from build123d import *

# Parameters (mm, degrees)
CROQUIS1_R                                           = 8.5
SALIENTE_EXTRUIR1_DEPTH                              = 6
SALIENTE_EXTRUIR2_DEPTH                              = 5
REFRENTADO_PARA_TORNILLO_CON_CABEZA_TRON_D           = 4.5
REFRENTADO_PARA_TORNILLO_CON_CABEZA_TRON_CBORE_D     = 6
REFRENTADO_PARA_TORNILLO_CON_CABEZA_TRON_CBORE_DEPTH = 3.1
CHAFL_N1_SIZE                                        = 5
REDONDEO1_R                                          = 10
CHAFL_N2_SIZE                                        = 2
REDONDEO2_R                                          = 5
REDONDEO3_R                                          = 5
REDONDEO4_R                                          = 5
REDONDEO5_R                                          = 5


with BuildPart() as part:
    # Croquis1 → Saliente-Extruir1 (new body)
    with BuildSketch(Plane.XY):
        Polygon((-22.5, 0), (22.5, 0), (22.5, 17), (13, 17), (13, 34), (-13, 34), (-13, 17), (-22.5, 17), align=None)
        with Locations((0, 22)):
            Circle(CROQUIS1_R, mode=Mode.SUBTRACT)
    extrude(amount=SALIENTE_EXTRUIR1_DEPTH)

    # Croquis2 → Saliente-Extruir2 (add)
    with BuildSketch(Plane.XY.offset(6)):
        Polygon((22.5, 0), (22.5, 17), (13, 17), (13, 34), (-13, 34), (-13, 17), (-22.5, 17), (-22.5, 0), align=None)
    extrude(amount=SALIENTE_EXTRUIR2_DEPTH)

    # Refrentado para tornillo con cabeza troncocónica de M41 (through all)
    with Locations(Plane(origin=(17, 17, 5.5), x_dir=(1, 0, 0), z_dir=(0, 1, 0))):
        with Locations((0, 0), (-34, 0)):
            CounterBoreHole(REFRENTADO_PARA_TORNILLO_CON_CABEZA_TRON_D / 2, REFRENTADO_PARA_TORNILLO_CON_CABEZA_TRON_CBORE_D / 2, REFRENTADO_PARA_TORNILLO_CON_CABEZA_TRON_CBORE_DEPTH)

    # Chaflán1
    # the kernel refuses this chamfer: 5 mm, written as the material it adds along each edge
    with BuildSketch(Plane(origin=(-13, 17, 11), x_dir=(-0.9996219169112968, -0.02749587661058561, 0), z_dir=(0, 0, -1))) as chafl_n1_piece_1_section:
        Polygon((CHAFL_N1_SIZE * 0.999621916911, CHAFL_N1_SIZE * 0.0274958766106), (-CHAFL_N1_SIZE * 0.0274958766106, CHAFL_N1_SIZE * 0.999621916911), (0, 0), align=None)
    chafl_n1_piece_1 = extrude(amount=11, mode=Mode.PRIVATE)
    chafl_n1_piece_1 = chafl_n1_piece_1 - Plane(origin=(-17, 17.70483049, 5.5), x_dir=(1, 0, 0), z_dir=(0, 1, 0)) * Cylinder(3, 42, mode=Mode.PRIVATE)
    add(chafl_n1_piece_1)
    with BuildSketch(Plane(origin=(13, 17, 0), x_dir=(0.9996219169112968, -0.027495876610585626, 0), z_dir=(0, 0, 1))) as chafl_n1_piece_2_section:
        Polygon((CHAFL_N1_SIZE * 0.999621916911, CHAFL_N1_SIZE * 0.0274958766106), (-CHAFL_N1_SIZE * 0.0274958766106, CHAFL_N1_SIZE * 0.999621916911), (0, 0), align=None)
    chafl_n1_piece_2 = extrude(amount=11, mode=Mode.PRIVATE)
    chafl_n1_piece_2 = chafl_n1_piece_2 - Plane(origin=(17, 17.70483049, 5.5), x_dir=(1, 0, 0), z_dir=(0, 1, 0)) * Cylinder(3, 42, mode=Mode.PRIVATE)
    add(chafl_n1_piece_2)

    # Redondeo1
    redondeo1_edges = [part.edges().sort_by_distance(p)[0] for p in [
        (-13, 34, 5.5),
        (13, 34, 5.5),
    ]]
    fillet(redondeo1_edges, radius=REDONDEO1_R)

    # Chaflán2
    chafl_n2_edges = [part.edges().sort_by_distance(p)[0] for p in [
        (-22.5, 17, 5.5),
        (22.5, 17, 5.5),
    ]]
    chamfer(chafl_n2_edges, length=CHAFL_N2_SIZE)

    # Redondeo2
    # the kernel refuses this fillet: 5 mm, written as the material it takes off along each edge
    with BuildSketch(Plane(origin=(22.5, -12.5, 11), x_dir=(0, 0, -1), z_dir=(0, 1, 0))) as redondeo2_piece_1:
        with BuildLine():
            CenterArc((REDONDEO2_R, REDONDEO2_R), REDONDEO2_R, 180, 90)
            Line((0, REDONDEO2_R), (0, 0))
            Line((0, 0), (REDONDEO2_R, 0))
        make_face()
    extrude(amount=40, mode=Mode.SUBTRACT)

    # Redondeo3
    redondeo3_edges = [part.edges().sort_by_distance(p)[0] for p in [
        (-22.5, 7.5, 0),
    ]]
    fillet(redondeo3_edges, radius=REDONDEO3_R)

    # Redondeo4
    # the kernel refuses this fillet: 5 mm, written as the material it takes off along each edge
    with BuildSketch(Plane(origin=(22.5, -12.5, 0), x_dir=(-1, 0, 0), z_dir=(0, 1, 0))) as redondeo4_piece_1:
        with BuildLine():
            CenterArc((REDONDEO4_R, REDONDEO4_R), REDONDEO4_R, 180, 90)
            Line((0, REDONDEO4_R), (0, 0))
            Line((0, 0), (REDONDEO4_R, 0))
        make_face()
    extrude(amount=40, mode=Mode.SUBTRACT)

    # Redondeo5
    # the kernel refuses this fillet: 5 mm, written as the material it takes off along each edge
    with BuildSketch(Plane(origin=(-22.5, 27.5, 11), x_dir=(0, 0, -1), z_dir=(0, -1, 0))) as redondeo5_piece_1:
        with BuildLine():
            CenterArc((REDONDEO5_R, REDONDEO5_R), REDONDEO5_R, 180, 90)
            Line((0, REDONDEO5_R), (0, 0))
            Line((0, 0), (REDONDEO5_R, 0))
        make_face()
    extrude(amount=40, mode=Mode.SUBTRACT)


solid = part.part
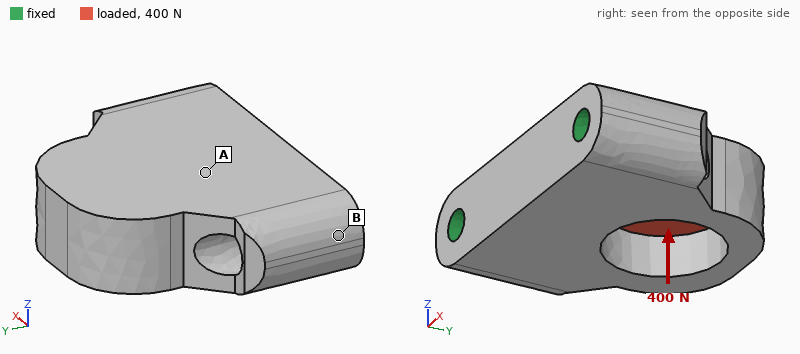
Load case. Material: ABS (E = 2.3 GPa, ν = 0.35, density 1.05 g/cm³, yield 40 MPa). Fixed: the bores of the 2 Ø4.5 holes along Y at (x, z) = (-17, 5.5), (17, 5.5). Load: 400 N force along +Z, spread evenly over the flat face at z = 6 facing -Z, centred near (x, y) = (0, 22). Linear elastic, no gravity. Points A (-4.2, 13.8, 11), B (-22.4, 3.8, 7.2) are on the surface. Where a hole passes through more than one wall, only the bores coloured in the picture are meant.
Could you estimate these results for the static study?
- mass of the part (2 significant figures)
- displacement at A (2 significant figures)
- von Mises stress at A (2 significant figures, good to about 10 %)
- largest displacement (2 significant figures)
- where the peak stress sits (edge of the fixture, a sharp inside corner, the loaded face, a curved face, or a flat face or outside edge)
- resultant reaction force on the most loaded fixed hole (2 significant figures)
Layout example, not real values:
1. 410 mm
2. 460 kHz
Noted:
1. 11 g
2. 0.076 mm
3. 5.7 MPa
4. 0.27 mm
5. edge of the fixture
6. 200 N
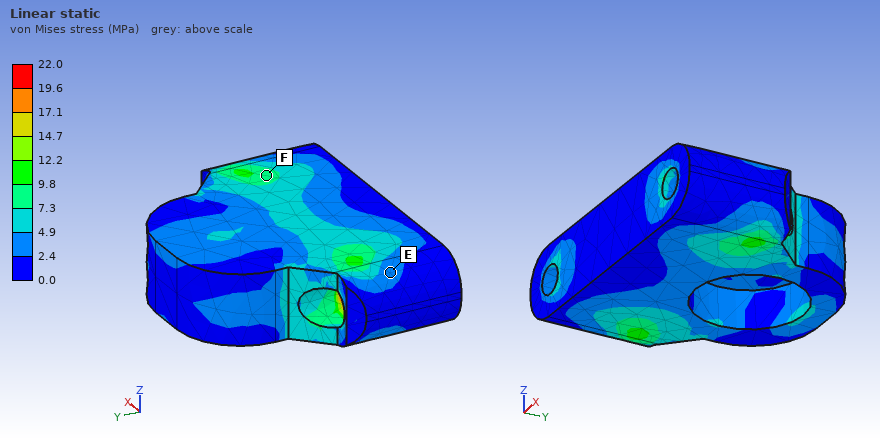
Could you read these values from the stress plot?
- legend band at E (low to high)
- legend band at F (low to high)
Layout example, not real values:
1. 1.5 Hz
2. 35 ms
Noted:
1. 2.4 to 4.9 MPa
2. 7.3 to 9.8 MPa
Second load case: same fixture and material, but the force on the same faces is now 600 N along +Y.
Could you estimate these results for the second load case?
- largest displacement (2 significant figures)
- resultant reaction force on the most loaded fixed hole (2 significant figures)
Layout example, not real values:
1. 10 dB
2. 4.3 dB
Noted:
1. 44 µm
2. 320 N
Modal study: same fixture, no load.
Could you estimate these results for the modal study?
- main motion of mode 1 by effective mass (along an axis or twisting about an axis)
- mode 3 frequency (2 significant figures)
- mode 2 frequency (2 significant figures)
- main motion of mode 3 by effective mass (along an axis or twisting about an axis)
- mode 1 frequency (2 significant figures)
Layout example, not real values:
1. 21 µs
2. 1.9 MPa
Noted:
1. along Z
2. 8900 Hz
3. 6700 Hz
4. along Z
5. 3400 Hz
